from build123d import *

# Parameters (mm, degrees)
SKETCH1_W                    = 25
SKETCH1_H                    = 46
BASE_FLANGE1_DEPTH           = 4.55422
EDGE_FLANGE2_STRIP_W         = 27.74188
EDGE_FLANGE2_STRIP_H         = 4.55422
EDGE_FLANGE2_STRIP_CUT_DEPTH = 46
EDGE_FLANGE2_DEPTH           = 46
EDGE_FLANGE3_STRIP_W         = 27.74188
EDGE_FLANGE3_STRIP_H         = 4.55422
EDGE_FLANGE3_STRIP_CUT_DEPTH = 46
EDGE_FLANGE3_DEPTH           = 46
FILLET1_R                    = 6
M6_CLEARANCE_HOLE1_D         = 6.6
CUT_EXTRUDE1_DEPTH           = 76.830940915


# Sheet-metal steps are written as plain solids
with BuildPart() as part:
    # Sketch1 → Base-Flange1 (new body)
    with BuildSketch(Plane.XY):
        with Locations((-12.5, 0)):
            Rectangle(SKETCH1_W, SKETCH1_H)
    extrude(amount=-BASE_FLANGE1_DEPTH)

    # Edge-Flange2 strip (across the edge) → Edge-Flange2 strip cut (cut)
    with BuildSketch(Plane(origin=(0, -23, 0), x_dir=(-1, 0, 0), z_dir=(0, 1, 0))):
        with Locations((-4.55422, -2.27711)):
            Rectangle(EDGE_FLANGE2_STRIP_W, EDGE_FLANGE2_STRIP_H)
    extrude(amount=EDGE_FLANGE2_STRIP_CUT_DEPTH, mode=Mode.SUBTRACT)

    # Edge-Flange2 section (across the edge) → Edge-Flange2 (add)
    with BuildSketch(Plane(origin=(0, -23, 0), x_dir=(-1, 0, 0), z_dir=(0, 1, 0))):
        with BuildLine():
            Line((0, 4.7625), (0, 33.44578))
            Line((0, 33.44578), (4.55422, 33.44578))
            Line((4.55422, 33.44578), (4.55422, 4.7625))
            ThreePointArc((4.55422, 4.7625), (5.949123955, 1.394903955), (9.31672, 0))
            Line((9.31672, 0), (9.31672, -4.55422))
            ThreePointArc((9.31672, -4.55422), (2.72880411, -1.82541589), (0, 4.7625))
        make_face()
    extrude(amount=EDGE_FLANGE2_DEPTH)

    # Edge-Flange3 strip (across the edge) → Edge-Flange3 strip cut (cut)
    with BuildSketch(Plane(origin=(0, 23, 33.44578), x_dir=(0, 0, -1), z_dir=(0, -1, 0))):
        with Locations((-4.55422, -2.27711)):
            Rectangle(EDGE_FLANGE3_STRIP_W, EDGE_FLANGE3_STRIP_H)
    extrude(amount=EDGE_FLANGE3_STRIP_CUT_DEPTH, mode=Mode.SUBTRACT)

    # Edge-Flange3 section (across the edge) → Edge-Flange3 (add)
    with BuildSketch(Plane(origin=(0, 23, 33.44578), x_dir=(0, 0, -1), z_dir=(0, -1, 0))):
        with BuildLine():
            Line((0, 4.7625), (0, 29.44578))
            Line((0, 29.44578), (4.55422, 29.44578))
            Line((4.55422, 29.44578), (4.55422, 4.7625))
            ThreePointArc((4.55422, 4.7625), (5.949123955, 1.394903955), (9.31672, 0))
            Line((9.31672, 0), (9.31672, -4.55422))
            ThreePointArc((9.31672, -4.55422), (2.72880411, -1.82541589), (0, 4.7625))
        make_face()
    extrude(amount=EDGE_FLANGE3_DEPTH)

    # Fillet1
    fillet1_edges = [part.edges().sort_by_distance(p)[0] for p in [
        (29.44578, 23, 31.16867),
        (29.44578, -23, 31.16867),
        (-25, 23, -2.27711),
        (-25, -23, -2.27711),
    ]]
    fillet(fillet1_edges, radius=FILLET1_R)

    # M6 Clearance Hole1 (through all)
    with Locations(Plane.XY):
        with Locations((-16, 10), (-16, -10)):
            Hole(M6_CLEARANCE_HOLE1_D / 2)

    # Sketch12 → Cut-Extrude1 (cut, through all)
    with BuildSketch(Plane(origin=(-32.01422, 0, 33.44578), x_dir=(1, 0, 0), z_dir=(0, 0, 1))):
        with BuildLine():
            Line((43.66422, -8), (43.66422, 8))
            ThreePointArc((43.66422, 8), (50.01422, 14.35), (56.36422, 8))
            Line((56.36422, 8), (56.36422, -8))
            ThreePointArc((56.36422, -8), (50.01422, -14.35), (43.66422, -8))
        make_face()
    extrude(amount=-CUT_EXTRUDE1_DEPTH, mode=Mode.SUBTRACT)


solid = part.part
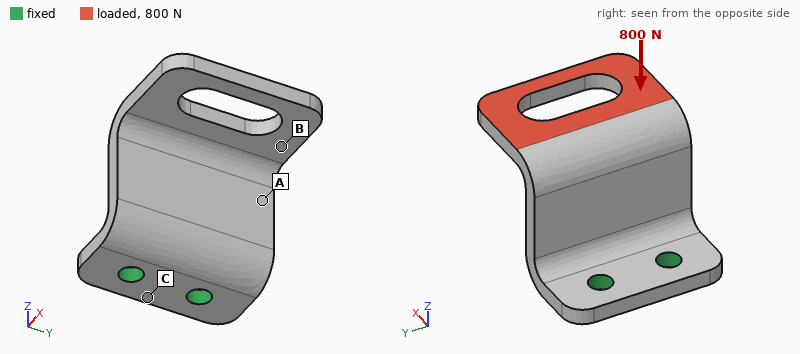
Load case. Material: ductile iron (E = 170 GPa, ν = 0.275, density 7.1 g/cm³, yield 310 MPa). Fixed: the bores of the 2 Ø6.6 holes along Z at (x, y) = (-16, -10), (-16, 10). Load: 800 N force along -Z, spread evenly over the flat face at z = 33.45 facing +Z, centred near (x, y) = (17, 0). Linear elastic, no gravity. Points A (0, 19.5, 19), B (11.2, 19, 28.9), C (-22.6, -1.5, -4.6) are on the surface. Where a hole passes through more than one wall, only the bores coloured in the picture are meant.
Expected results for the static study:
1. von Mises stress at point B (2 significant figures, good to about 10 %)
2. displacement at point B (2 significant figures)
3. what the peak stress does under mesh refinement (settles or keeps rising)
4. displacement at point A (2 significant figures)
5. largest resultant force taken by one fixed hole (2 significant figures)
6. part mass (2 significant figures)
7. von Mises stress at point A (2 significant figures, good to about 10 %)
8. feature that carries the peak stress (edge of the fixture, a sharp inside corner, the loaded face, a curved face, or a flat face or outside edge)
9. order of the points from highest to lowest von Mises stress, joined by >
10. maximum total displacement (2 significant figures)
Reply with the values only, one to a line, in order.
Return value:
62 MPa
0.28 mm
keeps rising
0.13 mm
410 N
110 g
97 MPa
edge of the fixture
A > B > C
0.52 mm
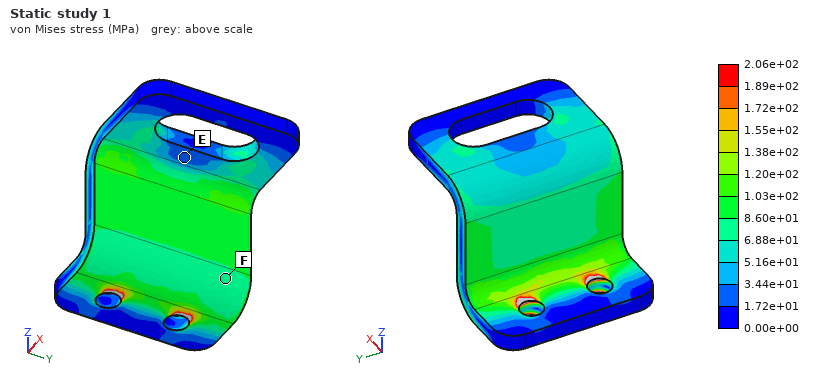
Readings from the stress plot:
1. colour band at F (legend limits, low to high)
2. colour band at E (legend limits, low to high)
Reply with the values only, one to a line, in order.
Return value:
6.88e+01 to 8.60e+01 MPa
1.72e+01 to 3.44e+01 MPa
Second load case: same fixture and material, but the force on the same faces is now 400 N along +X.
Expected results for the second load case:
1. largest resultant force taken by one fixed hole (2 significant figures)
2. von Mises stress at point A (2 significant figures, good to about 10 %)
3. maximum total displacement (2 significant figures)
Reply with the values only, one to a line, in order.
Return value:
210 N
36 MPa
0.28 mm
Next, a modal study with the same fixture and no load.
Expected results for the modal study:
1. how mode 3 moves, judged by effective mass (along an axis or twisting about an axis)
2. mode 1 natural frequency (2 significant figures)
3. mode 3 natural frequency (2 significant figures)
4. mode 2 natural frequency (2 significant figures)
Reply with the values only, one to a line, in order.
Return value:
along Y
1000 Hz
3300 Hz
2300 Hz
